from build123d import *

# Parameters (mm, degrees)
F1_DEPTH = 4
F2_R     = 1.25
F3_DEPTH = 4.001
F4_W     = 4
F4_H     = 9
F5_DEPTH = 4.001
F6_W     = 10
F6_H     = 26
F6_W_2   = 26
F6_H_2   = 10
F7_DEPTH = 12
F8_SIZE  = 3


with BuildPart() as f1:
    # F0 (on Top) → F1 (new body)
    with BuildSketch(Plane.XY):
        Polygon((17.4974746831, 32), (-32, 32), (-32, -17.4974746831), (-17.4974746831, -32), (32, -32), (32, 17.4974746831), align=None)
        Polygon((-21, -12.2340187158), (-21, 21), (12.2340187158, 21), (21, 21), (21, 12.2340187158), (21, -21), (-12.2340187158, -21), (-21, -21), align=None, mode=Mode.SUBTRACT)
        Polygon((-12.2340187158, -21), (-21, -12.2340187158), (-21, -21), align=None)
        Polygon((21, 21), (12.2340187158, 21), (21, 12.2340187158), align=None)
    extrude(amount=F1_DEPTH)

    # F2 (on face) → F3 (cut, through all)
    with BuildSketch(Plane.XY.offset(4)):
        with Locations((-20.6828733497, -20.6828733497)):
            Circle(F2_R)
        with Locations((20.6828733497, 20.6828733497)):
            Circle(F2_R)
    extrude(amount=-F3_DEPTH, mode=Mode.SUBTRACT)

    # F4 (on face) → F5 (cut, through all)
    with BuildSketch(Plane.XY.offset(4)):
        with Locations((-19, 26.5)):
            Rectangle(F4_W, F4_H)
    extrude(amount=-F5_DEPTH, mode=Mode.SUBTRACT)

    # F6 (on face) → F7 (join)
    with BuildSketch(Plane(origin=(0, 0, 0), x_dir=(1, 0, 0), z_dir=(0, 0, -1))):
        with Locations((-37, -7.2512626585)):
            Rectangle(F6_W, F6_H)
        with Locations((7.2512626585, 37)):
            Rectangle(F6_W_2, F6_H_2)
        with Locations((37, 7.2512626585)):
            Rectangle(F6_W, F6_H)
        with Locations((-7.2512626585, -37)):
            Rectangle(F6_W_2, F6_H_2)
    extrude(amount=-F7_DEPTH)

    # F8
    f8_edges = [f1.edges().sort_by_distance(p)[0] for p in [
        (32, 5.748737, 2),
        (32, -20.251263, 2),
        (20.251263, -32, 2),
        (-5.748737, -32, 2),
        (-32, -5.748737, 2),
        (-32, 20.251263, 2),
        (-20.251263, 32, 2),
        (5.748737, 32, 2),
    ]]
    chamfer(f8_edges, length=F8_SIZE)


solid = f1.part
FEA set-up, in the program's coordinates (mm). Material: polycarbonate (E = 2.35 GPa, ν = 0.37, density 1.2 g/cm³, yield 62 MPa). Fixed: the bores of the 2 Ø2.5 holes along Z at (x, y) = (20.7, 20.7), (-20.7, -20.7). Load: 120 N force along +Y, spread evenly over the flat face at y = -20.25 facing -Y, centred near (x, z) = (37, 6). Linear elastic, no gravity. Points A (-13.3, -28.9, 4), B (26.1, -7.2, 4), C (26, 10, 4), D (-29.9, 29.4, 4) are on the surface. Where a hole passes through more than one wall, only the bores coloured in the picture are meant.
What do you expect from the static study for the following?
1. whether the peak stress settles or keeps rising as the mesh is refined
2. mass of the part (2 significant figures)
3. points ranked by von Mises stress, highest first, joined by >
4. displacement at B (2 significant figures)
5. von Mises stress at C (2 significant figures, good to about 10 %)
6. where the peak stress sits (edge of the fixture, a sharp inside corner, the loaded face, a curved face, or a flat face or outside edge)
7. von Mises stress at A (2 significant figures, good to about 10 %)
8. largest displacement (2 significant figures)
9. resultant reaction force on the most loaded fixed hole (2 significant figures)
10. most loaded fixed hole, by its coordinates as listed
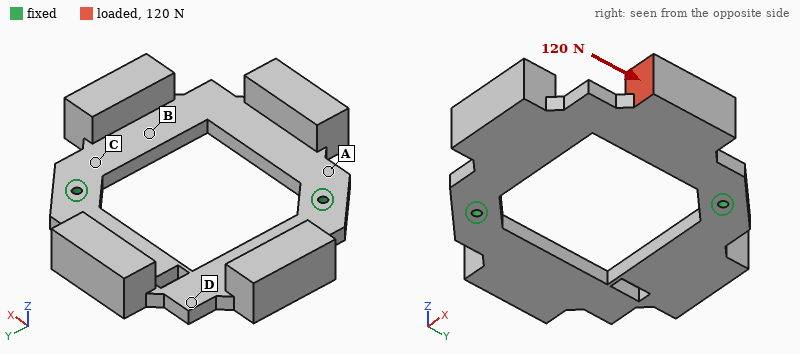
keeps rising
25 g
C > A > B > D
0.49 mm
10.0 MPa
edge of the fixture
5.7 MPa
1.2 mm
130 N
(20.7, 20.7)
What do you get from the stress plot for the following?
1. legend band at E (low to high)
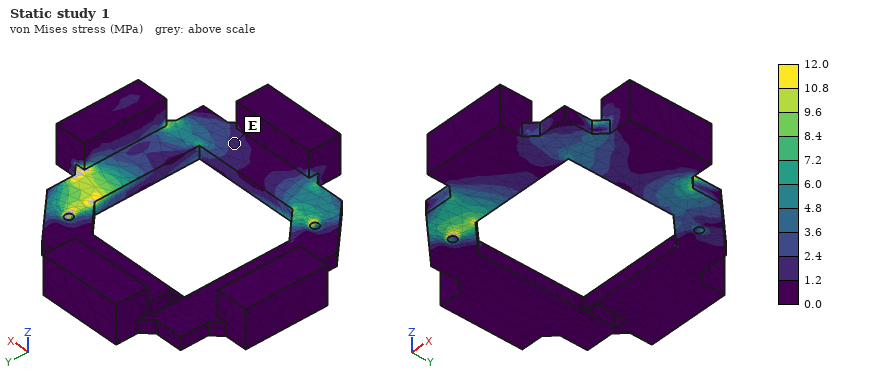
1.2 to 2.4 MPa
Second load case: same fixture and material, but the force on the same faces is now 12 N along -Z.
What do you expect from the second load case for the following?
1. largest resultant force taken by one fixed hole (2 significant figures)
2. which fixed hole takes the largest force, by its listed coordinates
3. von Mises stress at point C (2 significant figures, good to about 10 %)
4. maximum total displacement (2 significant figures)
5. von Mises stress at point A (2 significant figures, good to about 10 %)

8.0 N
(20.7, 20.7)
6.5 MPa
1.2 mm
5.3 MPa
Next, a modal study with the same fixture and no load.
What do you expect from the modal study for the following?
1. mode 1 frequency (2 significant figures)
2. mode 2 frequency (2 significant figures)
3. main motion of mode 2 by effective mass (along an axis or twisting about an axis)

240 Hz
250 Hz
along Z
